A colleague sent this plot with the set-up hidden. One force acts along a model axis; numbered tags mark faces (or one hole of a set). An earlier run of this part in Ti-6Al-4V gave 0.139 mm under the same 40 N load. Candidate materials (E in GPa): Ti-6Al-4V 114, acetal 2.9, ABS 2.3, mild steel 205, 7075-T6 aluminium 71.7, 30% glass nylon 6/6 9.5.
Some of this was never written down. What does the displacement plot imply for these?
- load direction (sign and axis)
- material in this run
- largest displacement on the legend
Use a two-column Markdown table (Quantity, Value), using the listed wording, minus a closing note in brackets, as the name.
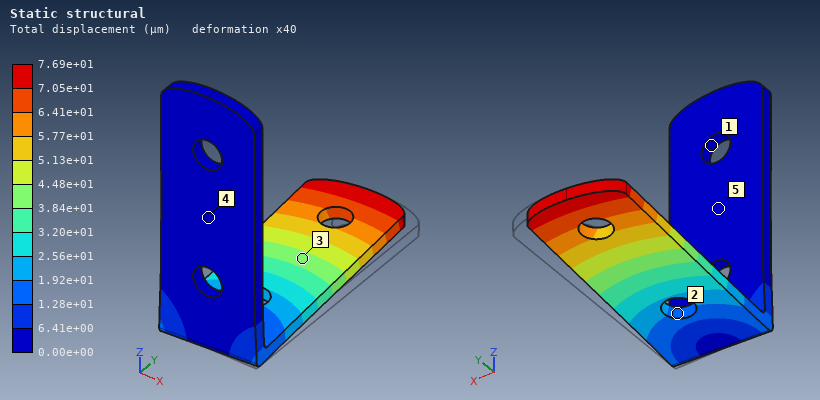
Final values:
| Quantity | Value |
|---|---|
| load direction | -X |
| material in this run | mild steel |
| largest displacement on the legend | 7.69e+01 µm |
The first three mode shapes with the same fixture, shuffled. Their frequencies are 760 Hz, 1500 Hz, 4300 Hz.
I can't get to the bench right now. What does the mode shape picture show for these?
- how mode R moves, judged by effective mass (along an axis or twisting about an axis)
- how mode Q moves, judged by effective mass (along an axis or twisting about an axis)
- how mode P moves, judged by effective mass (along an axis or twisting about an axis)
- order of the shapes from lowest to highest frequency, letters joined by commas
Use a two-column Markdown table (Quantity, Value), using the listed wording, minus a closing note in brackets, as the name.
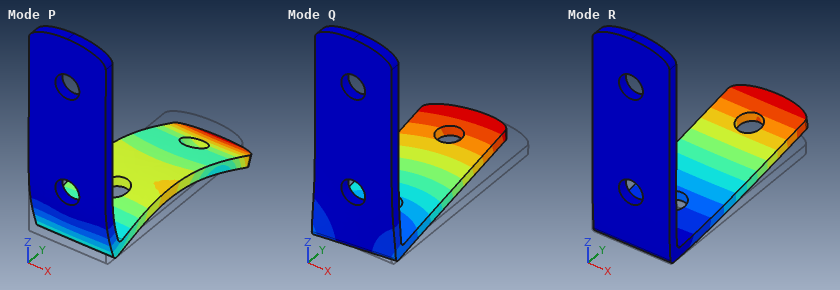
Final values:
| Quantity | Value |
|---|---|
| how mode R moves, judged by effective mass | along Z |
| how mode Q moves, judged by effective mass | along X |
| how mode P moves, judged by effective mass | along Y |
| order of the shapes from lowest to highest frequency, letters joined by commas | R, Q, P |
